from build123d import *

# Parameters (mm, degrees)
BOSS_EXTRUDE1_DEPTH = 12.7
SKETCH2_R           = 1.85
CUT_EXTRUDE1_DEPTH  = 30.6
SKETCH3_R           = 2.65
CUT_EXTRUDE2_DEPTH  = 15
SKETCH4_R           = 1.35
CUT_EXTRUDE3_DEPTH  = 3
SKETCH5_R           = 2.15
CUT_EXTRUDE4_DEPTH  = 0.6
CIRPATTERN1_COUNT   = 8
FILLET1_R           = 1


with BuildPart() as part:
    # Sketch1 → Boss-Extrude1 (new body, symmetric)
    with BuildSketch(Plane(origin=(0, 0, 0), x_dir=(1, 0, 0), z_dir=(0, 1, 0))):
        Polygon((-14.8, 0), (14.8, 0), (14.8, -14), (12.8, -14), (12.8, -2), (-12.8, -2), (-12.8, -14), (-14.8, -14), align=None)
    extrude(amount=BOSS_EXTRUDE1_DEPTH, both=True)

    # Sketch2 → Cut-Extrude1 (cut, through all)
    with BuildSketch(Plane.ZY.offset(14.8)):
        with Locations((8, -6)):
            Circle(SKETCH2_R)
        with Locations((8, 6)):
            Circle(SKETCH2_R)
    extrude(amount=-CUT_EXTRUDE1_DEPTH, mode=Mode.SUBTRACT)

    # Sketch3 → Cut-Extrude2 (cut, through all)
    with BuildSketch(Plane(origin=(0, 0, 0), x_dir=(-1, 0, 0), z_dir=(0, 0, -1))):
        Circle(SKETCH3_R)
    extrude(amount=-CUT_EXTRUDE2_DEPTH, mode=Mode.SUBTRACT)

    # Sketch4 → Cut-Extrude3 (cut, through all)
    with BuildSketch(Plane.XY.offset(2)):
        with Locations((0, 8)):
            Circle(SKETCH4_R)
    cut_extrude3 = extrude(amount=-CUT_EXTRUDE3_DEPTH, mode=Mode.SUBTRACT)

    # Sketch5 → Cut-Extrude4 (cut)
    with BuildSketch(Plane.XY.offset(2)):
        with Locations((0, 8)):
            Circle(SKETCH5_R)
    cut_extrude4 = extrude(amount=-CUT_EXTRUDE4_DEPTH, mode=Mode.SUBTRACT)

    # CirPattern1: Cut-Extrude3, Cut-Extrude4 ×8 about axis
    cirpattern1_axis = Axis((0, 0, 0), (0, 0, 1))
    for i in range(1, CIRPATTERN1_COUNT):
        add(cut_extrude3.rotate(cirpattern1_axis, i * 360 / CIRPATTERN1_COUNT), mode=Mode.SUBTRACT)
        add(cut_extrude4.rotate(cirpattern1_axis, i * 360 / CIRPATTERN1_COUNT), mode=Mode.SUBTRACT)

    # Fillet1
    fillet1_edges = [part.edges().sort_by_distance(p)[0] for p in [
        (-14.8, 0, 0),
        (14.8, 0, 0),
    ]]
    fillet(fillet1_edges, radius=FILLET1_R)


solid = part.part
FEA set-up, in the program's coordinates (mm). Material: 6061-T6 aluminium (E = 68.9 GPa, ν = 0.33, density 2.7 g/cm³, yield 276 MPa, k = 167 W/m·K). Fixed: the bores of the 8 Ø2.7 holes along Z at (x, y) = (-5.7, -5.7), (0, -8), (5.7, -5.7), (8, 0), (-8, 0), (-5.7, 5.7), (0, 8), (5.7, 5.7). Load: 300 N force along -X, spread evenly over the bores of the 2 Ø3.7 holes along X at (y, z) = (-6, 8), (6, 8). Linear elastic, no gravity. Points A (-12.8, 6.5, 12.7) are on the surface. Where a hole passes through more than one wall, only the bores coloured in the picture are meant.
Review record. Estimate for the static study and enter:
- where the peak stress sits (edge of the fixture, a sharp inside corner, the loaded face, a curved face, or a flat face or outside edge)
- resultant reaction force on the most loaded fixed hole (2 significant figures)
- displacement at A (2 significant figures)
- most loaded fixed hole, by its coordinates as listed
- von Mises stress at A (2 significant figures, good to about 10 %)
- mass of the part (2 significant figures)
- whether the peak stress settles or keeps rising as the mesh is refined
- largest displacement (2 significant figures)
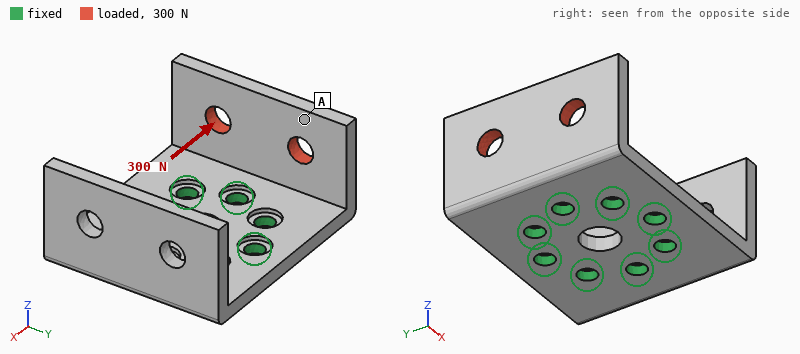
edge of the fixture
190 N
0.19 mm
(-8, 0)
20 MPa
6.6 g
keeps rising
0.23 mm
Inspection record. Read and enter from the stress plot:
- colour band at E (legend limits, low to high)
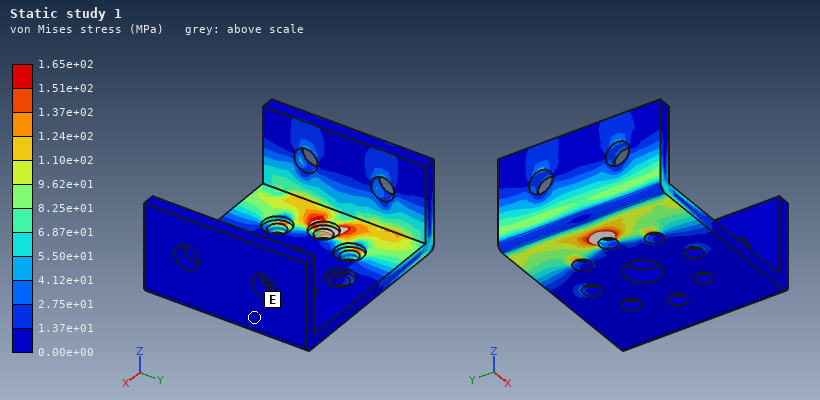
0.00e+00 to 1.37e+01 MPa
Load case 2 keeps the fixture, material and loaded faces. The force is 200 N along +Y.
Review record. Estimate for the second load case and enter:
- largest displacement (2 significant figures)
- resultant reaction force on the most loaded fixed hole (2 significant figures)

53 µm
130 N
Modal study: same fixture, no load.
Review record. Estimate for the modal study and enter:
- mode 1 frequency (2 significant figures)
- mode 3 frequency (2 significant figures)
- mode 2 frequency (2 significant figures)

5300 Hz
7600 Hz
5300 Hz
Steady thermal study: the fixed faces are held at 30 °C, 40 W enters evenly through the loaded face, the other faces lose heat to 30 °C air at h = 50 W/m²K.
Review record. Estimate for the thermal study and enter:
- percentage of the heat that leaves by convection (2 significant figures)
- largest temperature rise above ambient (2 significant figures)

5.9 %
73 K
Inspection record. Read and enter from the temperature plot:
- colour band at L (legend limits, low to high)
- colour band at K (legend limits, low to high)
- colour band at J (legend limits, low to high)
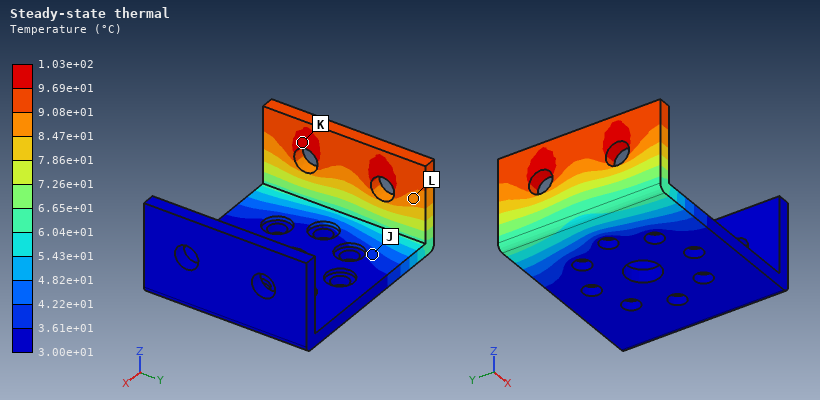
8.47e+01 to 9.08e+01 °C
9.69e+01 to 1.03e+02 °C
3.61e+01 to 4.22e+01 °C
